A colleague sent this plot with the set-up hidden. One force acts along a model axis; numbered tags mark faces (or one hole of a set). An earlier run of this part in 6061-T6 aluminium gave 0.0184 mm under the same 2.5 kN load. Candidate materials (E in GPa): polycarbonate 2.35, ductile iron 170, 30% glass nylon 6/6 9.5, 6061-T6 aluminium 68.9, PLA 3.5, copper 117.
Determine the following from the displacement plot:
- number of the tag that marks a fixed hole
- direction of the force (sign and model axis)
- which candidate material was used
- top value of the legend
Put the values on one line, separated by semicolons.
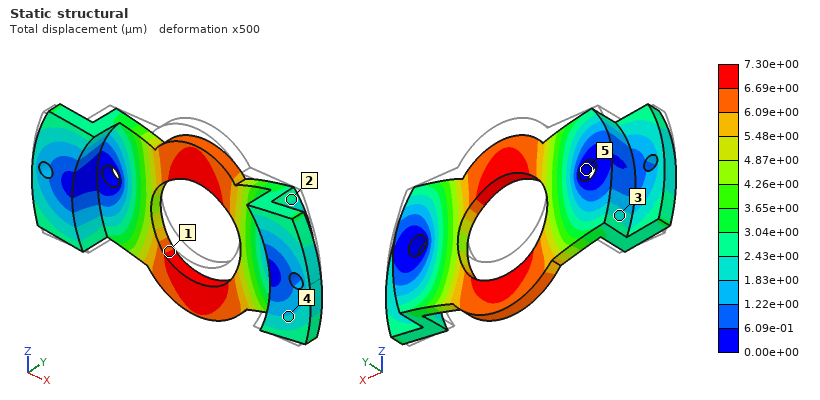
5; -Z; ductile iron; 7.30e+00 µm
